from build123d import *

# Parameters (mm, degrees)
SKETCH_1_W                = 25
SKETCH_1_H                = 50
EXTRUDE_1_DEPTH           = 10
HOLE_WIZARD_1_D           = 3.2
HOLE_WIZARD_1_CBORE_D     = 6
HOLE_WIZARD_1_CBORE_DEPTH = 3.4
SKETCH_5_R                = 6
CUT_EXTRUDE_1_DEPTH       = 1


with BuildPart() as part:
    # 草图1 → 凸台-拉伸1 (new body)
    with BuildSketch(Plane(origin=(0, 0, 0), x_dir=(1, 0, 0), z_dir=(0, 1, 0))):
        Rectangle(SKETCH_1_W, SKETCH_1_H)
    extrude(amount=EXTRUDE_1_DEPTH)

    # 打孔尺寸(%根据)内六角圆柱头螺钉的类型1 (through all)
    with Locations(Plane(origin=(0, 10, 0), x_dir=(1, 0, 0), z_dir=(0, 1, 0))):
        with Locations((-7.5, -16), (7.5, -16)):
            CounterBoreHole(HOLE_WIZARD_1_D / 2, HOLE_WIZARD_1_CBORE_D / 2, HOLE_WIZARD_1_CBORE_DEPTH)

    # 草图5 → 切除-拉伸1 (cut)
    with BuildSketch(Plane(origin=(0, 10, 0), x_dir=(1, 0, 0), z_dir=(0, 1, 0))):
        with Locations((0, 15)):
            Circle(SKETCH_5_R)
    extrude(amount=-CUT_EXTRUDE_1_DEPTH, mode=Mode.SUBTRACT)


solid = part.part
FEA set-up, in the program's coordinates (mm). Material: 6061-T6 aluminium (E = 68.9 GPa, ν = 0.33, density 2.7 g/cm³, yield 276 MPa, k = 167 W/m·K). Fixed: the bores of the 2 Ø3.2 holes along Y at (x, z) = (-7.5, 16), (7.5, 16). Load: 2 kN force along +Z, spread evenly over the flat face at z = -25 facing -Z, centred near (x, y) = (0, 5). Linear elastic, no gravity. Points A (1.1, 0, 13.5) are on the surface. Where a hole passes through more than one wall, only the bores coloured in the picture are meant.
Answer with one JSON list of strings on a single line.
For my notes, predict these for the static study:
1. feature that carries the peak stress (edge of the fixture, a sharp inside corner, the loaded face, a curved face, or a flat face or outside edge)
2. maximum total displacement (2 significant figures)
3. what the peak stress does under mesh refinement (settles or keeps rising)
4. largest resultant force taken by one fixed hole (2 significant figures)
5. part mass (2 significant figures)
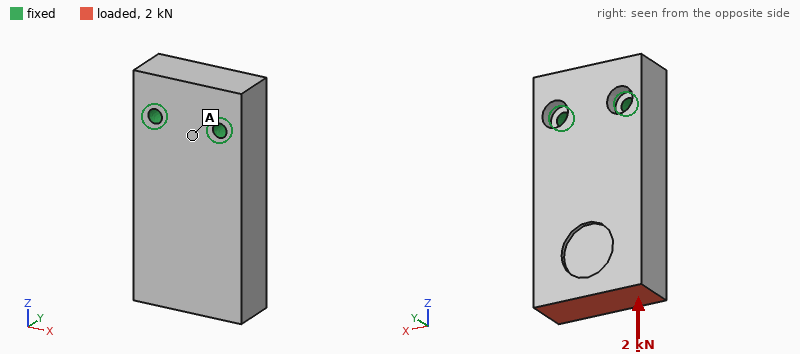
["edge of the fixture", "13 µm", "keeps rising", "1.0 kN", "33 g"]
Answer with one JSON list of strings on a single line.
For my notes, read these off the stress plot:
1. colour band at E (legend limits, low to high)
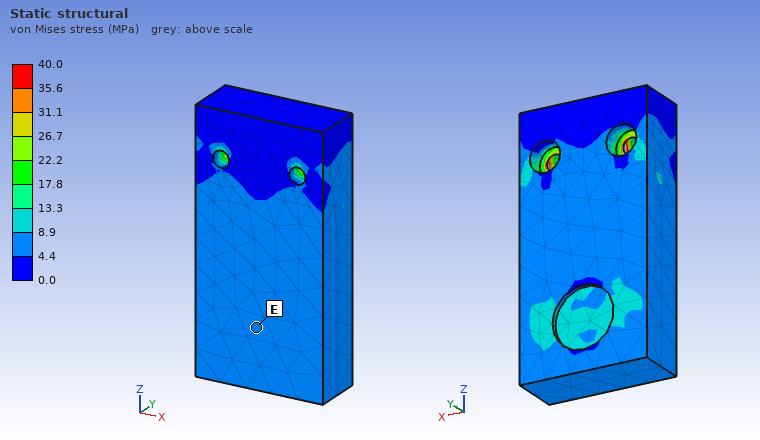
["4.4 to 8.9 MPa"]
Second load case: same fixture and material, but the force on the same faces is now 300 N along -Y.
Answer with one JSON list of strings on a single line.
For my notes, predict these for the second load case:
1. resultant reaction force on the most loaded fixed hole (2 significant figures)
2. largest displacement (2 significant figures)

["170 N", "76 µm"]
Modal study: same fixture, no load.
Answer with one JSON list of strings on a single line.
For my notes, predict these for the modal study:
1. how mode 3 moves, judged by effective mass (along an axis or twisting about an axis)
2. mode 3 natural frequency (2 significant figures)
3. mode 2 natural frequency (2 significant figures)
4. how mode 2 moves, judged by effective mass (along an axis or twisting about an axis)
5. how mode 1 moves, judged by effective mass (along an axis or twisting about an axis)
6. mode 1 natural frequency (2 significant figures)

["twisting about Z", "13 kHz", "8700 Hz", "along X", "along Y", "3700 Hz"]
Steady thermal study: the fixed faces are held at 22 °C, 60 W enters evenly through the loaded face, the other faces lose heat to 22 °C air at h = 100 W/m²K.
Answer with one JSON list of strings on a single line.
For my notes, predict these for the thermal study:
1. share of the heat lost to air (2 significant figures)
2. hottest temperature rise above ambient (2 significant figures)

["14 %", "57 K"]
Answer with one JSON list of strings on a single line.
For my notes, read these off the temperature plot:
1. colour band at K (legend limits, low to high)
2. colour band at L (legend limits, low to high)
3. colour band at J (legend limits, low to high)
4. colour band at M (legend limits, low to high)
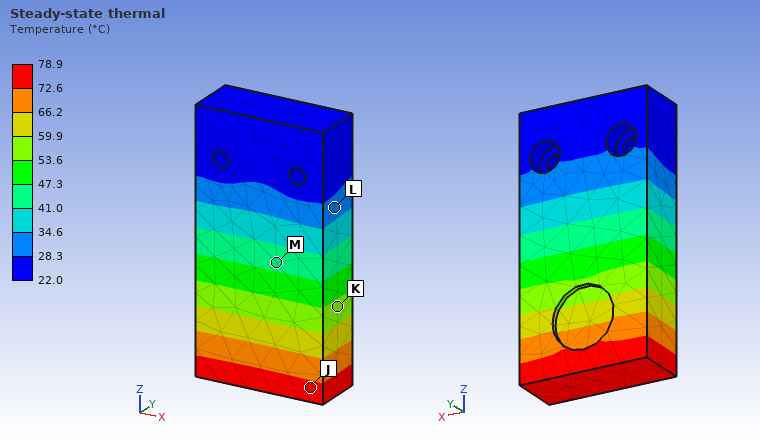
["53.6 to 59.9 °C", "28.3 to 34.6 °C", "72.6 to 78.9 °C", "41.0 to 47.3 °C"]
